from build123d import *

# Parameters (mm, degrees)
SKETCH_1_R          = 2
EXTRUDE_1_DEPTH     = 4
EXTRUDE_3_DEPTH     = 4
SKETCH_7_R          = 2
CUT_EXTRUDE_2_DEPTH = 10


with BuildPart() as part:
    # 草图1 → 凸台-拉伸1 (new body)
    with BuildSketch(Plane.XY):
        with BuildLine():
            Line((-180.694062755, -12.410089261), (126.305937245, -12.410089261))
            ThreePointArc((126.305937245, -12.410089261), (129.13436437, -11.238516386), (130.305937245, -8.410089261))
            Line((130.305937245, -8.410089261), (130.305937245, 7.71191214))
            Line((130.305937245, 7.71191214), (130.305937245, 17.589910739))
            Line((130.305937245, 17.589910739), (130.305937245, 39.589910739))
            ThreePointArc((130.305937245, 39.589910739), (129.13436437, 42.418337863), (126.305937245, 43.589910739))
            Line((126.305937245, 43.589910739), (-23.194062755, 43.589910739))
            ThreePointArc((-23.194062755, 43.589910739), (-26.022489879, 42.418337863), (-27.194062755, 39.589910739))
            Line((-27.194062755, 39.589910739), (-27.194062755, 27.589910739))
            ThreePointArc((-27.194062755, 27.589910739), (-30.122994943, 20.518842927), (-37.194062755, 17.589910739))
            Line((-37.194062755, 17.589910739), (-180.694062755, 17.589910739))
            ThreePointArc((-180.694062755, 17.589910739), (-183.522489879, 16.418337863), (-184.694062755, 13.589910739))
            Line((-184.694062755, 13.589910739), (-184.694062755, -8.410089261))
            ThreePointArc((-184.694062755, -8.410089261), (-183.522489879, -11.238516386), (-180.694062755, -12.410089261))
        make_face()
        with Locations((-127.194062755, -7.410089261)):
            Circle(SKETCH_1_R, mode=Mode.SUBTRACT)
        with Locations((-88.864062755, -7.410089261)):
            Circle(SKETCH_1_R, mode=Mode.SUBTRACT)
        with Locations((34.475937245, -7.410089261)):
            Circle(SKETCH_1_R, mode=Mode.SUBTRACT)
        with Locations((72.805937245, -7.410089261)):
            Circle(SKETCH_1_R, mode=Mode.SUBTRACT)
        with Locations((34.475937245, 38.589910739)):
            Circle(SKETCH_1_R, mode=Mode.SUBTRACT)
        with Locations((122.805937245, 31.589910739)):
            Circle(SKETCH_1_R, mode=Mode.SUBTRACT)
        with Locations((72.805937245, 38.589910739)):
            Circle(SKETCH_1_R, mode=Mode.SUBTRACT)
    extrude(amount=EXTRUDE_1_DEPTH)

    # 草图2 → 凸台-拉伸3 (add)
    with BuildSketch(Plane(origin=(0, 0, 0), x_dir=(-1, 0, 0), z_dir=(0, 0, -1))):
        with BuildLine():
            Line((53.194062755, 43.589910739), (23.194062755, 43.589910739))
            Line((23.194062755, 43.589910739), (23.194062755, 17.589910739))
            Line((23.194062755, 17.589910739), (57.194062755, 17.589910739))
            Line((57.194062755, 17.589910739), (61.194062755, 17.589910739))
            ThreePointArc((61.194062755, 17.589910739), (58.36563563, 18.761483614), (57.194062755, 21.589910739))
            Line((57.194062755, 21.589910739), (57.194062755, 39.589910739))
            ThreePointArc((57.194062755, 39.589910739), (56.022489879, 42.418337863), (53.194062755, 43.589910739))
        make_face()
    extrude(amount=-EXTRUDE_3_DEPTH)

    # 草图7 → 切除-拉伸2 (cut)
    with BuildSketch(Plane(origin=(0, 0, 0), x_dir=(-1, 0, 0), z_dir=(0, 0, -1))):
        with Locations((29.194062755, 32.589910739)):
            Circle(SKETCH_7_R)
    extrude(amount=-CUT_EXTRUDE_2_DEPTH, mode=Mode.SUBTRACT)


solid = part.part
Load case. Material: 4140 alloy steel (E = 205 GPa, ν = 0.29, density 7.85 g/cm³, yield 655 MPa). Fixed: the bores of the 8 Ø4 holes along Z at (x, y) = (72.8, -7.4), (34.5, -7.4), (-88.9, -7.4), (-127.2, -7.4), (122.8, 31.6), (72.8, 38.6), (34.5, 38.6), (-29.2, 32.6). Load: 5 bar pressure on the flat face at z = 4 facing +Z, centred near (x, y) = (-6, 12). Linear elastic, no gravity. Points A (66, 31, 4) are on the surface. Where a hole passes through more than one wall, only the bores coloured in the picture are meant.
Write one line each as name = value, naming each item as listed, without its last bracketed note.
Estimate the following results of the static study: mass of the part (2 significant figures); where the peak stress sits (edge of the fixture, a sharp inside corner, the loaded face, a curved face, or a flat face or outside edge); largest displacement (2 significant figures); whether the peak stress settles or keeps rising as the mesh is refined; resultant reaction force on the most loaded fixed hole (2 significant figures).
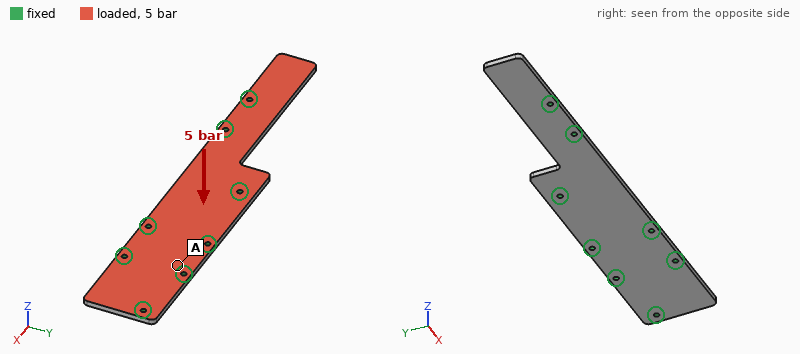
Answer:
mass of the part = 450 g
where the peak stress sits = edge of the fixture
largest displacement = 0.78 mm
whether the peak stress settles or keeps rising as the mesh is refined = keeps rising
resultant reaction force on the most loaded fixed hole = 1.5 kN
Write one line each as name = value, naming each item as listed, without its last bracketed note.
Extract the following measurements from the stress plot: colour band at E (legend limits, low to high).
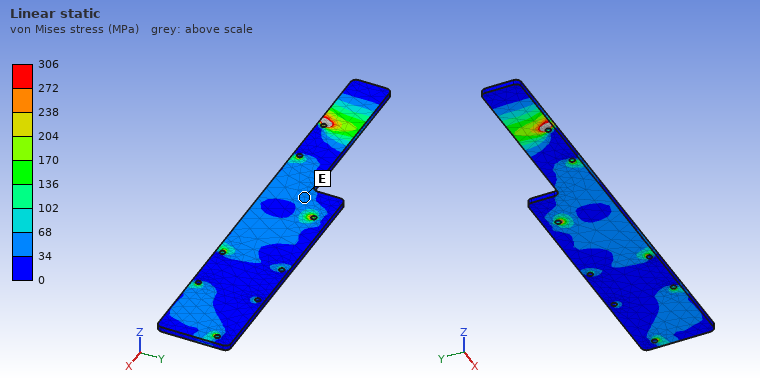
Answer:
colour band at E = 34 to 68 MPa
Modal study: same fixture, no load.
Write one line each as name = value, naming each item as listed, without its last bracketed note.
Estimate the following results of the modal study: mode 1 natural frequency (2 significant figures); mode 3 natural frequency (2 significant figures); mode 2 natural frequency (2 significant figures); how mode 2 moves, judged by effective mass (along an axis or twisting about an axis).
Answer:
mode 1 natural frequency = 910 Hz
mode 3 natural frequency = 2600 Hz
mode 2 natural frequency = 2300 Hz
how mode 2 moves, judged by effective mass = along Z
